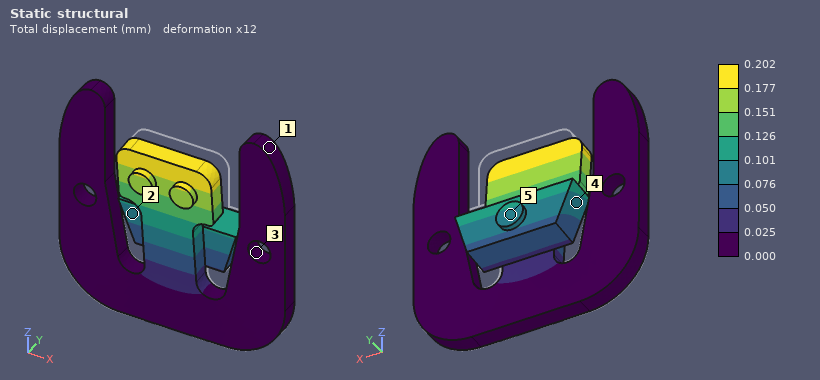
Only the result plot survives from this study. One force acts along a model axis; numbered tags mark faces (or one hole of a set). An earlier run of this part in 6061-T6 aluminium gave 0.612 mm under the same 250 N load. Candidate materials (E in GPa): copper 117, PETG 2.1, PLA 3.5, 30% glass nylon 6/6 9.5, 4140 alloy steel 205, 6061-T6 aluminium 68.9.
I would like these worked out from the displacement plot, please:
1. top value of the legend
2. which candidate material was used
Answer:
0.202 mm
4140 alloy steel
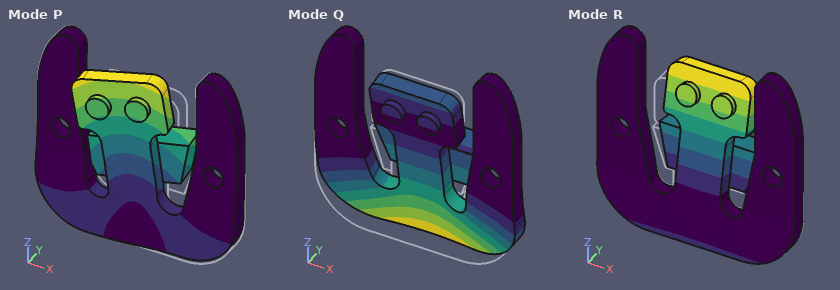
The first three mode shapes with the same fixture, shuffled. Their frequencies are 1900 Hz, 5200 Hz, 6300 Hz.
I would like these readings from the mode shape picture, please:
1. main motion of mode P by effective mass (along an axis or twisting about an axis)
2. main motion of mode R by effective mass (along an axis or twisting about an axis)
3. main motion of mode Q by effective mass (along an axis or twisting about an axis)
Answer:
along X
along Y
along Y
